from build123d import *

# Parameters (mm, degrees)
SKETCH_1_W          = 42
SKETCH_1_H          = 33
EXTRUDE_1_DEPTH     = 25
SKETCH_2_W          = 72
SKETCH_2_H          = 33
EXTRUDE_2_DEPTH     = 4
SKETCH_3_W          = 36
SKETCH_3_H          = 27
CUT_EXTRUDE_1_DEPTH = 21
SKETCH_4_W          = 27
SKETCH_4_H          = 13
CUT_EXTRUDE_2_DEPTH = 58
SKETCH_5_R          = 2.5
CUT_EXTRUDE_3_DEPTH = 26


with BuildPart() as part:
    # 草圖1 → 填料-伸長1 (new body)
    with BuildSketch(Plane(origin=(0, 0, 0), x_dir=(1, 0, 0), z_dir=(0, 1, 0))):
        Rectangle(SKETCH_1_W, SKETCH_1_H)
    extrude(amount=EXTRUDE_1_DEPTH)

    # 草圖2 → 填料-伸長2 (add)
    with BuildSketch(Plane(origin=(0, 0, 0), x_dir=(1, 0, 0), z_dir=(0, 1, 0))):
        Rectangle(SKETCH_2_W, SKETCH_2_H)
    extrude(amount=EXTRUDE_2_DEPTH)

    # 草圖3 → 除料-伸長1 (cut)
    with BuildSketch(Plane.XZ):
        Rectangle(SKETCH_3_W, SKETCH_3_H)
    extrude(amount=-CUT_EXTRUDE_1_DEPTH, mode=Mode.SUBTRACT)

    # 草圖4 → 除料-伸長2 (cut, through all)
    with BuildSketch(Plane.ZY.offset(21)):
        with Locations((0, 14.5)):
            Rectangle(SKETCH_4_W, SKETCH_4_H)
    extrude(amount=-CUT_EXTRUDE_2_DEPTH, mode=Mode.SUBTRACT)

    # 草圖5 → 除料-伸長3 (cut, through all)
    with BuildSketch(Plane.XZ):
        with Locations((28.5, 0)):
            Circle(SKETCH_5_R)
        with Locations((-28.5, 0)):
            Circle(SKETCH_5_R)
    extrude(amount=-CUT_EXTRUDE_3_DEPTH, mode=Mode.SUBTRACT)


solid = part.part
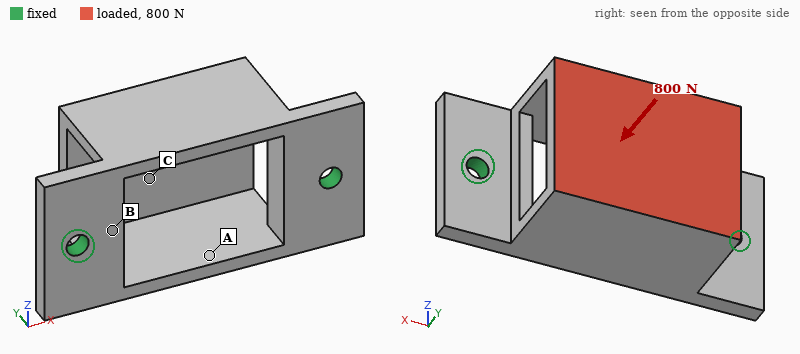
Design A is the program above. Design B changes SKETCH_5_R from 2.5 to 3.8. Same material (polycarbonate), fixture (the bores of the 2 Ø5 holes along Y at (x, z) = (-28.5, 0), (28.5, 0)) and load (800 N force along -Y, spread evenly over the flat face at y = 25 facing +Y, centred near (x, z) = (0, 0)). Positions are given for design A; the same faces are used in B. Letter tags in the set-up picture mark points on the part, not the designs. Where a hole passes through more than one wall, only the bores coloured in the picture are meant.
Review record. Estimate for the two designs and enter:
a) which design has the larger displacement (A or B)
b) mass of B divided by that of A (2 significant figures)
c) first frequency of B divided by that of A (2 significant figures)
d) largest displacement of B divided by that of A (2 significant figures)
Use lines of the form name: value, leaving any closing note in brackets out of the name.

which design has the larger displacement: A
mass of B divided by that of A: 0.99
first frequency of B divided by that of A: 1.1
largest displacement of B divided by that of A: 0.88
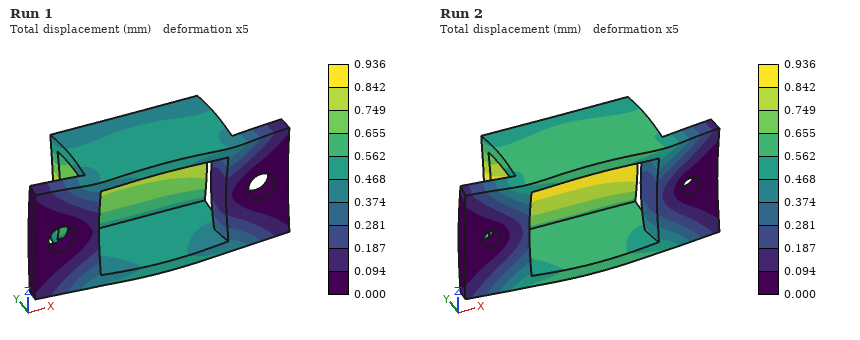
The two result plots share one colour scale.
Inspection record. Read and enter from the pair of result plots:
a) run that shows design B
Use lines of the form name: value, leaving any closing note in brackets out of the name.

run that shows design B: Run 1
